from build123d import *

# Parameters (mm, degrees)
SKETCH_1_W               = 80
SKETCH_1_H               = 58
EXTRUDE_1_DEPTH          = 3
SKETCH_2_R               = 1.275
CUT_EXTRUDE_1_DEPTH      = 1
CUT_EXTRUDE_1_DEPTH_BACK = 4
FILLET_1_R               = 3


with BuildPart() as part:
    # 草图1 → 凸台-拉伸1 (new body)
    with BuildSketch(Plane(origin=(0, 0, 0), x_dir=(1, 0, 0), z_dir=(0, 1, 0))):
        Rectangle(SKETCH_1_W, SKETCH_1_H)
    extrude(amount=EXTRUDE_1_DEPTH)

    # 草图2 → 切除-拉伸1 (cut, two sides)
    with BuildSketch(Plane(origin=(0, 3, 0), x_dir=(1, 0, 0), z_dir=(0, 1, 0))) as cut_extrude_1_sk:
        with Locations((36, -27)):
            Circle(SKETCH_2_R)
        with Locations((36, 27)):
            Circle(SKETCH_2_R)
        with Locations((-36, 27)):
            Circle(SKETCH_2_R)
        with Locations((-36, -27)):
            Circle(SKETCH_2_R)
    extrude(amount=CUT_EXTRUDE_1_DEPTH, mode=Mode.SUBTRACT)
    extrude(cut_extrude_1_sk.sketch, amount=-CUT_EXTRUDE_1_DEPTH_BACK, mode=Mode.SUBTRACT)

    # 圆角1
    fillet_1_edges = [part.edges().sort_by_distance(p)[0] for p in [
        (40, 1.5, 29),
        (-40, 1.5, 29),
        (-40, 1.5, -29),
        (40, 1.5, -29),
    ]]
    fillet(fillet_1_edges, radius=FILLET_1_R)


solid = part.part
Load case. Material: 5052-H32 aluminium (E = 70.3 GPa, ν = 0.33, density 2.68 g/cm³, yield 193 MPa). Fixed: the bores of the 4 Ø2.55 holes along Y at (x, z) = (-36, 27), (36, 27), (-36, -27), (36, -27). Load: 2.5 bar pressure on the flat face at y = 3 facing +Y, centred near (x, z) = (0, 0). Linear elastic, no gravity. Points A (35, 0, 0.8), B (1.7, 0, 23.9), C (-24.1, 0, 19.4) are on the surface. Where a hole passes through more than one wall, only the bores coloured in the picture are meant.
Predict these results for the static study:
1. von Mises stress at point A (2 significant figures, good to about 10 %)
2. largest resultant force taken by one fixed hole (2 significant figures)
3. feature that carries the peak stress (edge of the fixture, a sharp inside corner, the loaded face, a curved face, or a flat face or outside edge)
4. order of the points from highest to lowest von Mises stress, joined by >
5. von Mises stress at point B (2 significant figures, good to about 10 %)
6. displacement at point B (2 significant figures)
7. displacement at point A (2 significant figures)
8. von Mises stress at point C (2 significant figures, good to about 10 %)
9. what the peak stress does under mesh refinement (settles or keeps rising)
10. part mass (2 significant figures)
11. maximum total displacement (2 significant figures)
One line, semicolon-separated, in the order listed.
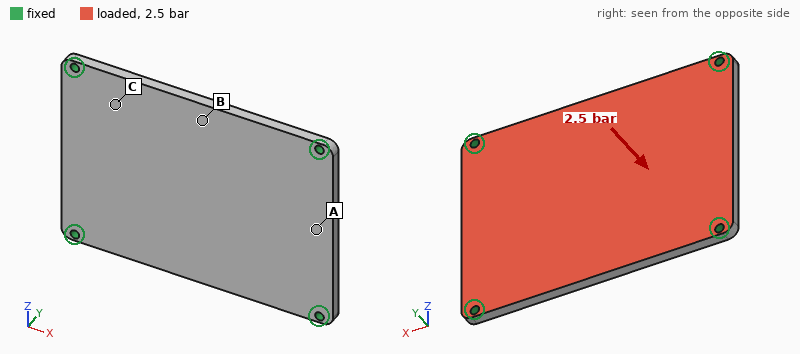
33 MPa; 290 N; edge of the fixture; B > A > C; 52 MPa; 0.20 mm; 0.071 mm; 15 MPa; keeps rising; 37 g; 0.23 mm
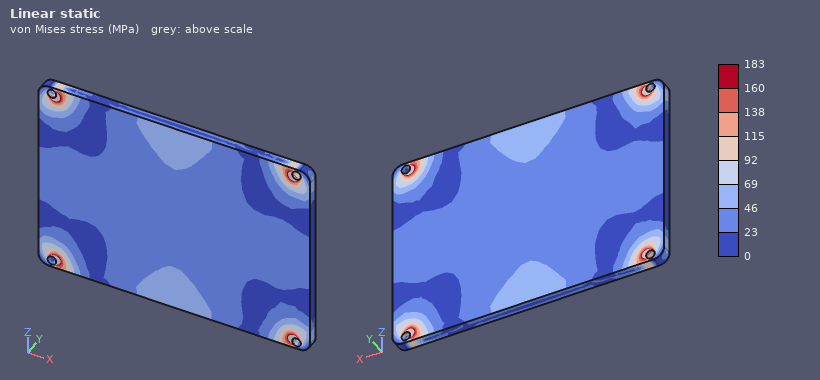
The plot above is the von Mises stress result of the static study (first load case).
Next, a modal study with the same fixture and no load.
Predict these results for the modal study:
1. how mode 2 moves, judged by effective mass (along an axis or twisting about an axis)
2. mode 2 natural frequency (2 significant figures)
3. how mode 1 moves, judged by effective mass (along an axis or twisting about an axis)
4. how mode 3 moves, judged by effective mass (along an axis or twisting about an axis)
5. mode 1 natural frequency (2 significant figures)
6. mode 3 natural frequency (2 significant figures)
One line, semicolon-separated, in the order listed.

twisting about X; 3700 Hz; along Y; twisting about Z; 2200 Hz; 4900 Hz
